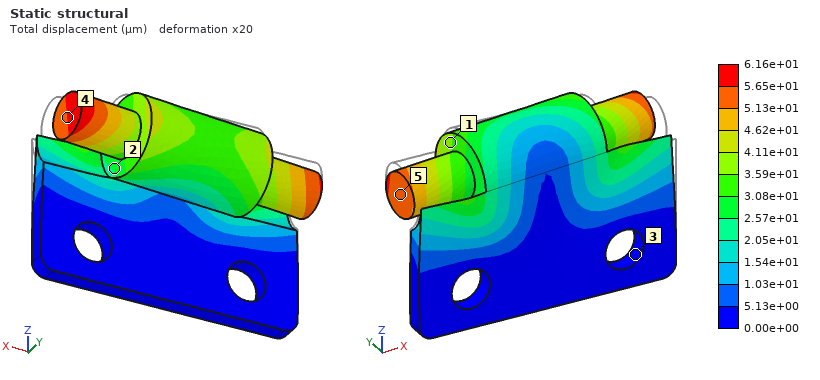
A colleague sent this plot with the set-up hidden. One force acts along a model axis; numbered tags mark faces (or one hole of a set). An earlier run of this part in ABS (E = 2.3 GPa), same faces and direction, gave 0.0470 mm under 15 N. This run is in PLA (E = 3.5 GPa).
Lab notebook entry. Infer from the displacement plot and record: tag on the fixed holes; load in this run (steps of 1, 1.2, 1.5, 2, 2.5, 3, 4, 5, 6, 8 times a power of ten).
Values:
3
30 N
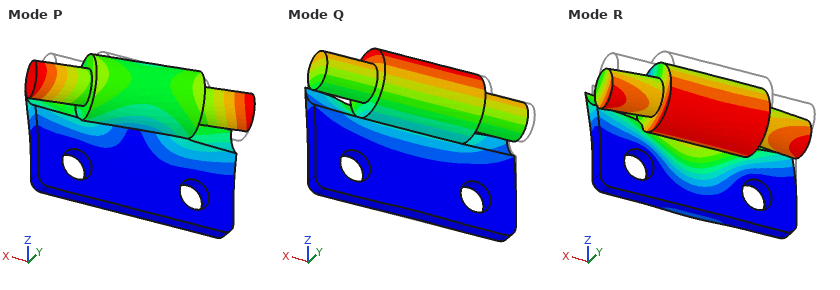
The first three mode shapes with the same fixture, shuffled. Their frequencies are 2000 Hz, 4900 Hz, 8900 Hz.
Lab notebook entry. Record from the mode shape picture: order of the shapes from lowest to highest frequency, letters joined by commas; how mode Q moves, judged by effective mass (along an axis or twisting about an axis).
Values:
Q, P, R
along Y
